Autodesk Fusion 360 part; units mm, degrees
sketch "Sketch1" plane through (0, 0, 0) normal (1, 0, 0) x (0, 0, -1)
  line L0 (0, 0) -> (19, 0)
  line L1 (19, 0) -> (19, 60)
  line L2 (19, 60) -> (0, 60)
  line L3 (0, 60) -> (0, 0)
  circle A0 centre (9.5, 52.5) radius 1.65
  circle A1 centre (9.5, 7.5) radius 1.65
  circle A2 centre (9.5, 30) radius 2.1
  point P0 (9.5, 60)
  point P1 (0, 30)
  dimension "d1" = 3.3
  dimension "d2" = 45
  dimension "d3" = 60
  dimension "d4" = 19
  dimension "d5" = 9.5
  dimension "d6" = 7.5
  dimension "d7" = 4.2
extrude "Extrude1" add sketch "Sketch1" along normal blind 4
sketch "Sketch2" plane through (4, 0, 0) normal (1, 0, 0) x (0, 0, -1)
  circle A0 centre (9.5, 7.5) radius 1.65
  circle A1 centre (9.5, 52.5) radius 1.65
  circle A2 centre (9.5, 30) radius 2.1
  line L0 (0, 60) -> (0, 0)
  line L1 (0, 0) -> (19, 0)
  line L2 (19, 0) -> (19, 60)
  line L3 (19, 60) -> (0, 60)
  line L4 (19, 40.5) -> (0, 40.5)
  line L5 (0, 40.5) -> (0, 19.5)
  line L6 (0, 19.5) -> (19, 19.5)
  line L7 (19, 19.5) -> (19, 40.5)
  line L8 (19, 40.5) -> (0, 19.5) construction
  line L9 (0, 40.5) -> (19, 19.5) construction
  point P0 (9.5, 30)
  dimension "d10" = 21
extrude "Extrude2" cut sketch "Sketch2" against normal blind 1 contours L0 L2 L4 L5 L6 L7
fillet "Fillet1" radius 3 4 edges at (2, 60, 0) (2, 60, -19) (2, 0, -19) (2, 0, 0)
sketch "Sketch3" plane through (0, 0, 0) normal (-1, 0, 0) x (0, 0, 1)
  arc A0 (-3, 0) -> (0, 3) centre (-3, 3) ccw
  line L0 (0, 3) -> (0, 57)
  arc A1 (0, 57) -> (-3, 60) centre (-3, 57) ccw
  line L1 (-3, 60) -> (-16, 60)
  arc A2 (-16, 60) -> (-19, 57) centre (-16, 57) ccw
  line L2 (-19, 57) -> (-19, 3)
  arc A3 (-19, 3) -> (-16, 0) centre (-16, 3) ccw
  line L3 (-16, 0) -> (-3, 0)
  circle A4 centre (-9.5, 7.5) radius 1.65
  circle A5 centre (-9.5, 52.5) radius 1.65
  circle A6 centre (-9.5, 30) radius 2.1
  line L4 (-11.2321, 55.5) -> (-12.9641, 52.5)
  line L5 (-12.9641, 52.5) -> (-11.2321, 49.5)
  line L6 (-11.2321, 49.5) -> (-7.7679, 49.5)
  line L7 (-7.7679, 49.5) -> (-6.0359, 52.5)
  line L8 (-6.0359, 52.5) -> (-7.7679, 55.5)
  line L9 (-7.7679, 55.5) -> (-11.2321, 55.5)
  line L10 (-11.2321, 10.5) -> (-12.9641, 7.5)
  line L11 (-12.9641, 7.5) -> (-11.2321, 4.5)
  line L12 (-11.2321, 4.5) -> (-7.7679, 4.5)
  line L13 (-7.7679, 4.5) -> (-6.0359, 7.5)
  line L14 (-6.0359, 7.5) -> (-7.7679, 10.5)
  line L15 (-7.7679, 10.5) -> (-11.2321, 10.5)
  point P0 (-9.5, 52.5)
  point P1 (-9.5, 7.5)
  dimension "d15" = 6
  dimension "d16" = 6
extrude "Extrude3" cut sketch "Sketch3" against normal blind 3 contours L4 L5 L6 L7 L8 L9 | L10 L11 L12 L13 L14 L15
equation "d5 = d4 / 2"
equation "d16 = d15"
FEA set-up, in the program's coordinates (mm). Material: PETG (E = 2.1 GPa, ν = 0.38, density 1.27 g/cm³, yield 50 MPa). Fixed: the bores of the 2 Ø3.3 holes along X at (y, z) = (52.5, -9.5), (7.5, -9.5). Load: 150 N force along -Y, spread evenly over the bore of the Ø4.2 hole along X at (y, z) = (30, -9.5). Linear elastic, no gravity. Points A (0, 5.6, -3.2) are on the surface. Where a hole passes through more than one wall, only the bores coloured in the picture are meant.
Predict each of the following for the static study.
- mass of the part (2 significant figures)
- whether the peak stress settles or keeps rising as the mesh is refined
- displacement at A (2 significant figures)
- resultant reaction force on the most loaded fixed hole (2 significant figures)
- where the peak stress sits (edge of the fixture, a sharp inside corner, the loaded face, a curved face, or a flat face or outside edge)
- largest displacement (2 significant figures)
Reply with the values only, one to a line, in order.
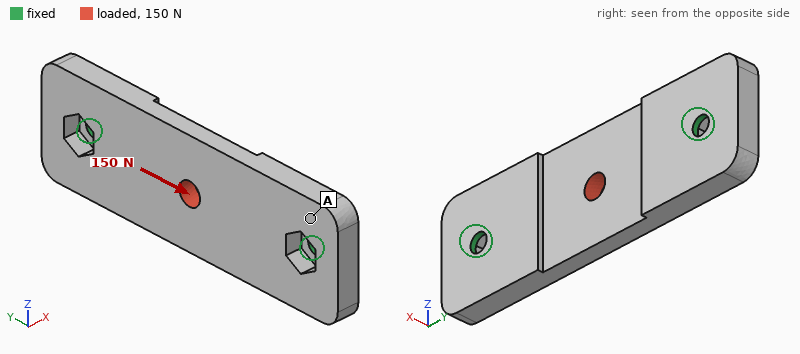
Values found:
4.9 g
keeps rising
24 µm
75 N
edge of the fixture
37 µm
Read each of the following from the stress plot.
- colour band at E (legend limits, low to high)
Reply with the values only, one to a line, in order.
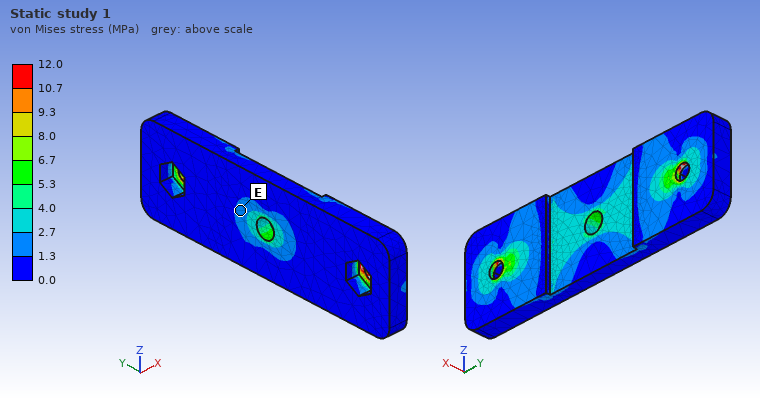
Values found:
1.3 to 2.7 MPa
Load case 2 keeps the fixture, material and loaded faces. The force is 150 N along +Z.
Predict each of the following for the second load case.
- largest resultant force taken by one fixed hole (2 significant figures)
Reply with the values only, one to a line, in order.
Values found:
75 N
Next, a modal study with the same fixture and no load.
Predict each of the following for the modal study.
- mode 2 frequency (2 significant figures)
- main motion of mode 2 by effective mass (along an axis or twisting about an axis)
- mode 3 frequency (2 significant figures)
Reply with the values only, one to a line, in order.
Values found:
1700 Hz
along X
2700 Hz
